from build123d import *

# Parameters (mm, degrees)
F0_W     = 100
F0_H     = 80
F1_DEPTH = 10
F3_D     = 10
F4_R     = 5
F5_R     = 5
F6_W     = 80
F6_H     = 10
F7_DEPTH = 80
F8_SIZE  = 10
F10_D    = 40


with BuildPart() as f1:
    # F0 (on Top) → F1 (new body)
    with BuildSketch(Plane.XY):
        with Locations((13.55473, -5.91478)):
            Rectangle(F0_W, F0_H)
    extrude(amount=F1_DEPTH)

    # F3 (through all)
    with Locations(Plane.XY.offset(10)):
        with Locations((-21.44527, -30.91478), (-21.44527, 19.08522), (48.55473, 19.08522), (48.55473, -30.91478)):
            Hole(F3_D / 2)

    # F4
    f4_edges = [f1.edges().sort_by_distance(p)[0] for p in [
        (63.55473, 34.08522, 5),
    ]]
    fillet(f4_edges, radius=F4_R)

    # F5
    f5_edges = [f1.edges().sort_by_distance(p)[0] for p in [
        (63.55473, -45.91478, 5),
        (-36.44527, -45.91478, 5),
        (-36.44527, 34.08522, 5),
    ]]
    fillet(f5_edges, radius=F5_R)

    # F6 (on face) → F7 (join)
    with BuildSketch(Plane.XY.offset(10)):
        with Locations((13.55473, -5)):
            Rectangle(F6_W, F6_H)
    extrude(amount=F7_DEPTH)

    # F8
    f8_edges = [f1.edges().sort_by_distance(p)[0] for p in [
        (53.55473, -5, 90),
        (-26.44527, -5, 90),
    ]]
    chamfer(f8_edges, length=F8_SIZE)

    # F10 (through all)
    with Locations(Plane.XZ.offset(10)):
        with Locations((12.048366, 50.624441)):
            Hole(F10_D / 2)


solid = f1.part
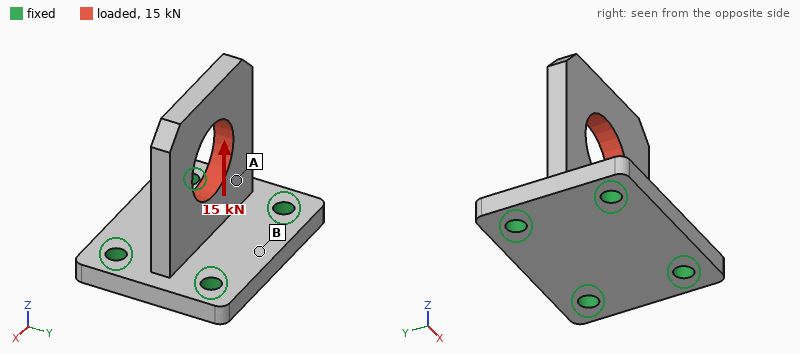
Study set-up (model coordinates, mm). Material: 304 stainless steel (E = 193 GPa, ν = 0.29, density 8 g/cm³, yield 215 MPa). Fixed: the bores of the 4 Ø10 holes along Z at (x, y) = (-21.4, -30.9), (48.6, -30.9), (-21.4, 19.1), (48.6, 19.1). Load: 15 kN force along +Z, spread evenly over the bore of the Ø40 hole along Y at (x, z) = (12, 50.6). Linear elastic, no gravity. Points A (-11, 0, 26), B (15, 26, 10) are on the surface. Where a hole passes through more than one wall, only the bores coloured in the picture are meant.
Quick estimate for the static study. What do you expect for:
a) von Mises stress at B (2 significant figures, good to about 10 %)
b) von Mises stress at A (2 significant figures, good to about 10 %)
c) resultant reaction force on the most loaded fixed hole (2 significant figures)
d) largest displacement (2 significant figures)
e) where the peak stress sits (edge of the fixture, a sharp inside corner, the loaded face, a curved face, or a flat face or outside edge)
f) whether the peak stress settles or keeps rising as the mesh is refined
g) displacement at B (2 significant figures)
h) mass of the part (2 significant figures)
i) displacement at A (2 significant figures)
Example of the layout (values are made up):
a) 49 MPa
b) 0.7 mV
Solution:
a) 9.7 MPa
b) 24 MPa
c) 4.2 kN
d) 21 µm
e) edge of the fixture
f) keeps rising
g) 3.3 µm
h) 1.0 kg
i) 11 µm
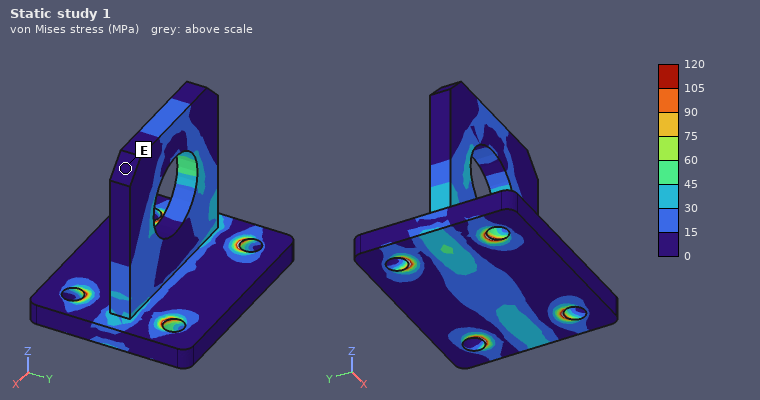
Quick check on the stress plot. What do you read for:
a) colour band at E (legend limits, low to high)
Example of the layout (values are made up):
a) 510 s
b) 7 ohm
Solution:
a) 0 to 15 MPa
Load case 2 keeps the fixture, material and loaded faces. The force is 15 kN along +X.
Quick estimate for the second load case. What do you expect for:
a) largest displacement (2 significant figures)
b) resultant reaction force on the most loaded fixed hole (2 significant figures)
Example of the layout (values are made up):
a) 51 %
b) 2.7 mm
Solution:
a) 83 µm
b) 6.6 kN
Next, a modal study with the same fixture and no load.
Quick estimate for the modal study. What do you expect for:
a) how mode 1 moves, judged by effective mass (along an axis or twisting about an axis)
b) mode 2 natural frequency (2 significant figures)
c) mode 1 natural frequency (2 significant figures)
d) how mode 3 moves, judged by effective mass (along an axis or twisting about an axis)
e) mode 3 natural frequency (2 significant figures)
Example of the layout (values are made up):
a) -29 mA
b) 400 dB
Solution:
a) along Y
b) 2500 Hz
c) 1100 Hz
d) along X
e) 3800 Hz
